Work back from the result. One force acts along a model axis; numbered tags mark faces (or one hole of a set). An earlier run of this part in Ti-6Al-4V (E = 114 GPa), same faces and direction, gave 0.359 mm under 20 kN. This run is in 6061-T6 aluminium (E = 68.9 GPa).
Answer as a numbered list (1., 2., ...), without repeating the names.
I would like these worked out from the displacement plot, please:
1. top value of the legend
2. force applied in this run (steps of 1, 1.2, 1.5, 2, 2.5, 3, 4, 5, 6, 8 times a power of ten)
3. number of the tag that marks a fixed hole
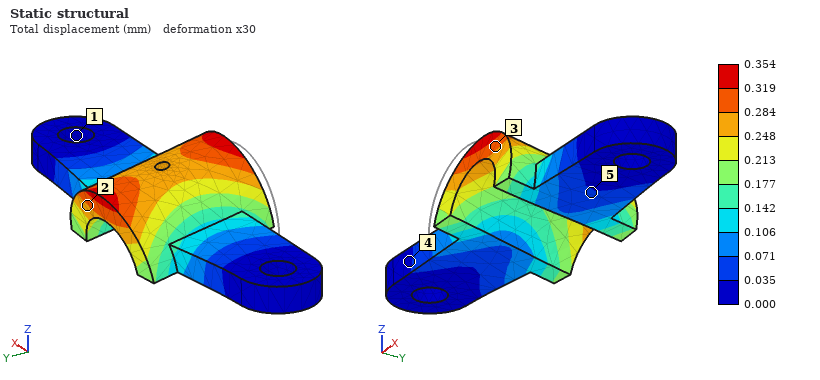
1. 0.354 mm
2. 12 kN
3. 1
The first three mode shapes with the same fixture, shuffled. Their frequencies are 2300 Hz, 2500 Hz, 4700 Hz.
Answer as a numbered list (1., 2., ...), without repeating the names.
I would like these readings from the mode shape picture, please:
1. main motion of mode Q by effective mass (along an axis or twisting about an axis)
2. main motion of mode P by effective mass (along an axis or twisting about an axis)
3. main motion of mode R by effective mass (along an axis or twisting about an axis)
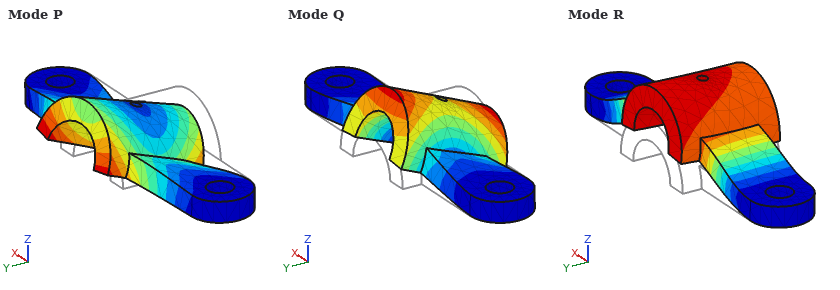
1. along Y
2. along Y
3. along Z
